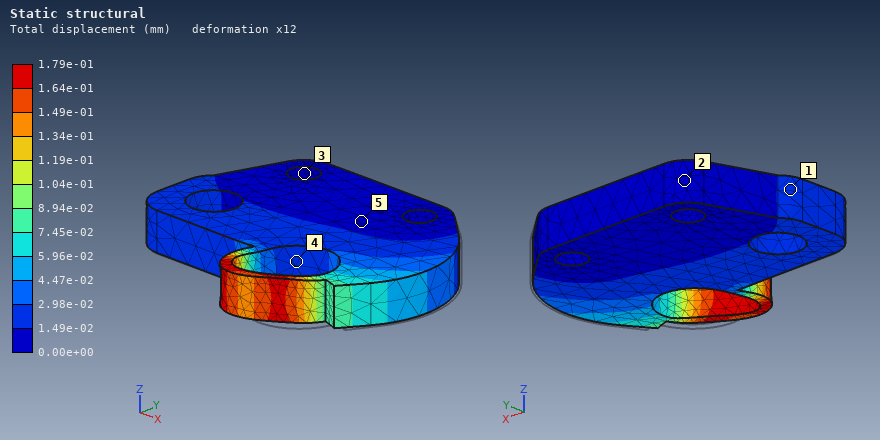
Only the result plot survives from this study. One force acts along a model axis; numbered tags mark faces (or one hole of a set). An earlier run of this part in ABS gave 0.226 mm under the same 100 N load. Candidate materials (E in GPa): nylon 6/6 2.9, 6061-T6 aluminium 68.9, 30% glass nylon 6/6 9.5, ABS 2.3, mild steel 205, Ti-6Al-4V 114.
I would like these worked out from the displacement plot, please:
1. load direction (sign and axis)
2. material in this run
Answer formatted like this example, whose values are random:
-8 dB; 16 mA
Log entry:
-X; nylon 6/6
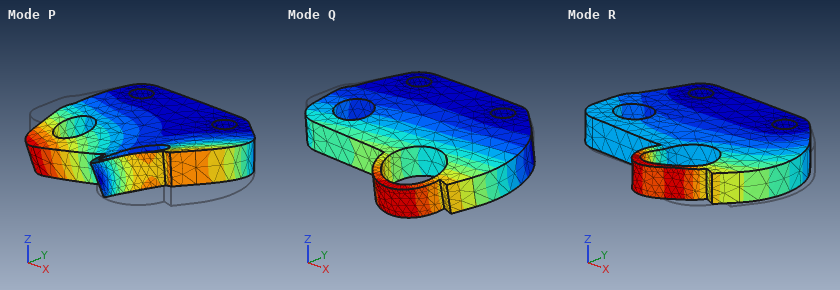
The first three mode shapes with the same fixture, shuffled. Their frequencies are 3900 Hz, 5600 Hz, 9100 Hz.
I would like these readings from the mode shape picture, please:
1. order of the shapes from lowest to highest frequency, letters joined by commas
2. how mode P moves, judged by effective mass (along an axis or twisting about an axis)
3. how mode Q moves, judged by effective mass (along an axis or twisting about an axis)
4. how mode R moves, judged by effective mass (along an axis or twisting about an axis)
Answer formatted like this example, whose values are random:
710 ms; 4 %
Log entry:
Q, P, R; twisting about Y; along Z; along X
